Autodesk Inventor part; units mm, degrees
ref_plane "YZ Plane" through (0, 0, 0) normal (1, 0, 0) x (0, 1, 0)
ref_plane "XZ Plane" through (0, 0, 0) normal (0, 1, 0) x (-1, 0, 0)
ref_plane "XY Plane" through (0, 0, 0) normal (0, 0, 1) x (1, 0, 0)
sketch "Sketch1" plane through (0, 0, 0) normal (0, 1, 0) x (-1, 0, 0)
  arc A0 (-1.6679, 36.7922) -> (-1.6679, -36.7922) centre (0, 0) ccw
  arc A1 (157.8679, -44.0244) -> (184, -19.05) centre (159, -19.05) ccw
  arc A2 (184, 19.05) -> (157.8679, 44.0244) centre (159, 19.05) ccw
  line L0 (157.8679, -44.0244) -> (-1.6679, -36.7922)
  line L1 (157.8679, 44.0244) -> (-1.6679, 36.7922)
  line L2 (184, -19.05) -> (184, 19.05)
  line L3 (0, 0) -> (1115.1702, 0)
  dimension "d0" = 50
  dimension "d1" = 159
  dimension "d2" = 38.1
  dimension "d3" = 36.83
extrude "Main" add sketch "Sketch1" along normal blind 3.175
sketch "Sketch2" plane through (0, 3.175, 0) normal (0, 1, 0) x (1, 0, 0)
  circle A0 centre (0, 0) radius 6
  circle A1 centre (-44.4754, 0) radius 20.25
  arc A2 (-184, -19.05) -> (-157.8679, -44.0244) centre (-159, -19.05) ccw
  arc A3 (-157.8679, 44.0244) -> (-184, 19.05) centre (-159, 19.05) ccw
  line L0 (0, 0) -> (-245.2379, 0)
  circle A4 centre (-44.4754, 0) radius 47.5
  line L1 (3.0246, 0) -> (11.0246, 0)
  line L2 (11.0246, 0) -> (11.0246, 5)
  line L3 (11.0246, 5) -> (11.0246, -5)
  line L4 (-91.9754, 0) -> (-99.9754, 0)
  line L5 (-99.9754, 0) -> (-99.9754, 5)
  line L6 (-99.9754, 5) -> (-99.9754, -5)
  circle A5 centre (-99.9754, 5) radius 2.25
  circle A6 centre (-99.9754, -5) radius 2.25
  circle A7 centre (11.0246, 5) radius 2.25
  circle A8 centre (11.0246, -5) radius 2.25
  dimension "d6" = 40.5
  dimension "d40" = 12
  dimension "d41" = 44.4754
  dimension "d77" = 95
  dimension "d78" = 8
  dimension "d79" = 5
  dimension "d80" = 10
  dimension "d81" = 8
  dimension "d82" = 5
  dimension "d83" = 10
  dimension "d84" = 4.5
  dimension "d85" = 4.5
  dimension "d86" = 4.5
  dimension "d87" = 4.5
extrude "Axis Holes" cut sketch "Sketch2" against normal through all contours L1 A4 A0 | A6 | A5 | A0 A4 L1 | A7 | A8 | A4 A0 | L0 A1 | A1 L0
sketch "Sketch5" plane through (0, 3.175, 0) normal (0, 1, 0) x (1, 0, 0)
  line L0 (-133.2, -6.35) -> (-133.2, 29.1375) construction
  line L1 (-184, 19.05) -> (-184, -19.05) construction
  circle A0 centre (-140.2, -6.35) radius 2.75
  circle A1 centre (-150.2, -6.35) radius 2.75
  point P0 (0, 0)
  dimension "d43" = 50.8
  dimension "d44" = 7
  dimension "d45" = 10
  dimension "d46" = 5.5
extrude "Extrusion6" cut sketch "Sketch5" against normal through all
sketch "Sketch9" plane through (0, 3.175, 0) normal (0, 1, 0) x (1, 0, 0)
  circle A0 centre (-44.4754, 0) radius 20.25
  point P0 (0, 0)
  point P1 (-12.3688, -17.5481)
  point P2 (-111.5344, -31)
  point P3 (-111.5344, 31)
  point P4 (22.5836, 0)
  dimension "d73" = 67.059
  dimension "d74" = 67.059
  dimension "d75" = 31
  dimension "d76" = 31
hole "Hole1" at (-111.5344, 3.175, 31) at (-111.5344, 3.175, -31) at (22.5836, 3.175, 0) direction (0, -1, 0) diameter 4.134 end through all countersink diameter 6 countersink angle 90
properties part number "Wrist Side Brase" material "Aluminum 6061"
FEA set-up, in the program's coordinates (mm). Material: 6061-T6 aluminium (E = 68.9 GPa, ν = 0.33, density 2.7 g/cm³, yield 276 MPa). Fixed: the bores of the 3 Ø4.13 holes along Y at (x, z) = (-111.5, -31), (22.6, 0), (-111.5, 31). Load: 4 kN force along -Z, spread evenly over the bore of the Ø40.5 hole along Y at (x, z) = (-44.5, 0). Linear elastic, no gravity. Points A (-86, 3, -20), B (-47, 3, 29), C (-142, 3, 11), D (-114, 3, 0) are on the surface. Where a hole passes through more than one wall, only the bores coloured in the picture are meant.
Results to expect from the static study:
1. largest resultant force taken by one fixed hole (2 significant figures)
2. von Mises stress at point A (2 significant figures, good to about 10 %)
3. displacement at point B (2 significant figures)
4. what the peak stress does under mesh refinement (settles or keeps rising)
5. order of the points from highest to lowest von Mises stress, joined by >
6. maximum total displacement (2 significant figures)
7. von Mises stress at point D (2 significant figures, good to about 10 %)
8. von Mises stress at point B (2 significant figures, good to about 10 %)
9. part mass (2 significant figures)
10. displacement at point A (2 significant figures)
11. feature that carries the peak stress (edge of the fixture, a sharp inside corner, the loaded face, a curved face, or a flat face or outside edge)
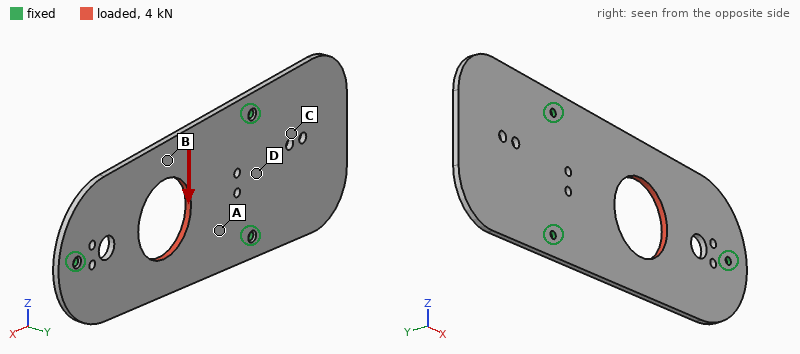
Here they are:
1.6 kN
18 MPa
40 µm
keeps rising
B > A > D > C
46 µm
7.8 MPa
25 MPa
130 g
16 µm
edge of the fixture
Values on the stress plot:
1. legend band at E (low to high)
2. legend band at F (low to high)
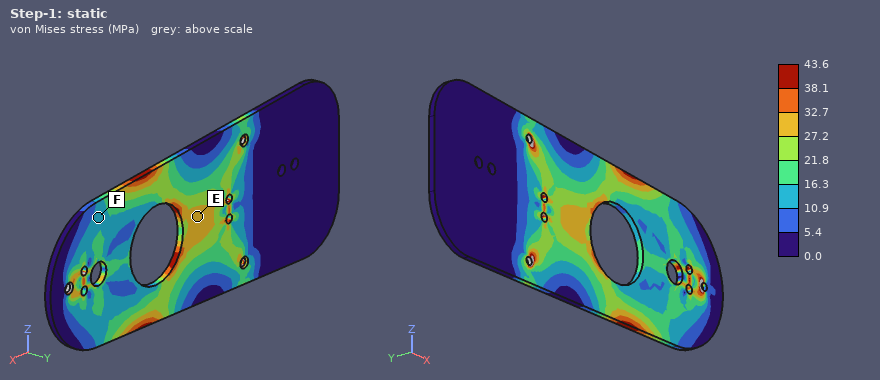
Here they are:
27.2 to 32.7 MPa
10.9 to 16.3 MPa
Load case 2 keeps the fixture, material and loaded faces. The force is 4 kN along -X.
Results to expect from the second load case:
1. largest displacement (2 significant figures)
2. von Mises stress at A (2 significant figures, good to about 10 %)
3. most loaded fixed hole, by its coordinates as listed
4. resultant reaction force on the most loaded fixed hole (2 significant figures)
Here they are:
15 µm
10 MPa
(22.6, 0)
1.5 kN
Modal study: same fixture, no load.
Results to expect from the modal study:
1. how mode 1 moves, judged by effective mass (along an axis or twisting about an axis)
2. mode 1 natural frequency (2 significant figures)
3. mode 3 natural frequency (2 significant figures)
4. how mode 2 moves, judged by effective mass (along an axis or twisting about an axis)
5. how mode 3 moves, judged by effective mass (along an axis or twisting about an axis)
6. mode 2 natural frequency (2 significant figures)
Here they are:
along Y
460 Hz
970 Hz
along Y
twisting about X
790 Hz
